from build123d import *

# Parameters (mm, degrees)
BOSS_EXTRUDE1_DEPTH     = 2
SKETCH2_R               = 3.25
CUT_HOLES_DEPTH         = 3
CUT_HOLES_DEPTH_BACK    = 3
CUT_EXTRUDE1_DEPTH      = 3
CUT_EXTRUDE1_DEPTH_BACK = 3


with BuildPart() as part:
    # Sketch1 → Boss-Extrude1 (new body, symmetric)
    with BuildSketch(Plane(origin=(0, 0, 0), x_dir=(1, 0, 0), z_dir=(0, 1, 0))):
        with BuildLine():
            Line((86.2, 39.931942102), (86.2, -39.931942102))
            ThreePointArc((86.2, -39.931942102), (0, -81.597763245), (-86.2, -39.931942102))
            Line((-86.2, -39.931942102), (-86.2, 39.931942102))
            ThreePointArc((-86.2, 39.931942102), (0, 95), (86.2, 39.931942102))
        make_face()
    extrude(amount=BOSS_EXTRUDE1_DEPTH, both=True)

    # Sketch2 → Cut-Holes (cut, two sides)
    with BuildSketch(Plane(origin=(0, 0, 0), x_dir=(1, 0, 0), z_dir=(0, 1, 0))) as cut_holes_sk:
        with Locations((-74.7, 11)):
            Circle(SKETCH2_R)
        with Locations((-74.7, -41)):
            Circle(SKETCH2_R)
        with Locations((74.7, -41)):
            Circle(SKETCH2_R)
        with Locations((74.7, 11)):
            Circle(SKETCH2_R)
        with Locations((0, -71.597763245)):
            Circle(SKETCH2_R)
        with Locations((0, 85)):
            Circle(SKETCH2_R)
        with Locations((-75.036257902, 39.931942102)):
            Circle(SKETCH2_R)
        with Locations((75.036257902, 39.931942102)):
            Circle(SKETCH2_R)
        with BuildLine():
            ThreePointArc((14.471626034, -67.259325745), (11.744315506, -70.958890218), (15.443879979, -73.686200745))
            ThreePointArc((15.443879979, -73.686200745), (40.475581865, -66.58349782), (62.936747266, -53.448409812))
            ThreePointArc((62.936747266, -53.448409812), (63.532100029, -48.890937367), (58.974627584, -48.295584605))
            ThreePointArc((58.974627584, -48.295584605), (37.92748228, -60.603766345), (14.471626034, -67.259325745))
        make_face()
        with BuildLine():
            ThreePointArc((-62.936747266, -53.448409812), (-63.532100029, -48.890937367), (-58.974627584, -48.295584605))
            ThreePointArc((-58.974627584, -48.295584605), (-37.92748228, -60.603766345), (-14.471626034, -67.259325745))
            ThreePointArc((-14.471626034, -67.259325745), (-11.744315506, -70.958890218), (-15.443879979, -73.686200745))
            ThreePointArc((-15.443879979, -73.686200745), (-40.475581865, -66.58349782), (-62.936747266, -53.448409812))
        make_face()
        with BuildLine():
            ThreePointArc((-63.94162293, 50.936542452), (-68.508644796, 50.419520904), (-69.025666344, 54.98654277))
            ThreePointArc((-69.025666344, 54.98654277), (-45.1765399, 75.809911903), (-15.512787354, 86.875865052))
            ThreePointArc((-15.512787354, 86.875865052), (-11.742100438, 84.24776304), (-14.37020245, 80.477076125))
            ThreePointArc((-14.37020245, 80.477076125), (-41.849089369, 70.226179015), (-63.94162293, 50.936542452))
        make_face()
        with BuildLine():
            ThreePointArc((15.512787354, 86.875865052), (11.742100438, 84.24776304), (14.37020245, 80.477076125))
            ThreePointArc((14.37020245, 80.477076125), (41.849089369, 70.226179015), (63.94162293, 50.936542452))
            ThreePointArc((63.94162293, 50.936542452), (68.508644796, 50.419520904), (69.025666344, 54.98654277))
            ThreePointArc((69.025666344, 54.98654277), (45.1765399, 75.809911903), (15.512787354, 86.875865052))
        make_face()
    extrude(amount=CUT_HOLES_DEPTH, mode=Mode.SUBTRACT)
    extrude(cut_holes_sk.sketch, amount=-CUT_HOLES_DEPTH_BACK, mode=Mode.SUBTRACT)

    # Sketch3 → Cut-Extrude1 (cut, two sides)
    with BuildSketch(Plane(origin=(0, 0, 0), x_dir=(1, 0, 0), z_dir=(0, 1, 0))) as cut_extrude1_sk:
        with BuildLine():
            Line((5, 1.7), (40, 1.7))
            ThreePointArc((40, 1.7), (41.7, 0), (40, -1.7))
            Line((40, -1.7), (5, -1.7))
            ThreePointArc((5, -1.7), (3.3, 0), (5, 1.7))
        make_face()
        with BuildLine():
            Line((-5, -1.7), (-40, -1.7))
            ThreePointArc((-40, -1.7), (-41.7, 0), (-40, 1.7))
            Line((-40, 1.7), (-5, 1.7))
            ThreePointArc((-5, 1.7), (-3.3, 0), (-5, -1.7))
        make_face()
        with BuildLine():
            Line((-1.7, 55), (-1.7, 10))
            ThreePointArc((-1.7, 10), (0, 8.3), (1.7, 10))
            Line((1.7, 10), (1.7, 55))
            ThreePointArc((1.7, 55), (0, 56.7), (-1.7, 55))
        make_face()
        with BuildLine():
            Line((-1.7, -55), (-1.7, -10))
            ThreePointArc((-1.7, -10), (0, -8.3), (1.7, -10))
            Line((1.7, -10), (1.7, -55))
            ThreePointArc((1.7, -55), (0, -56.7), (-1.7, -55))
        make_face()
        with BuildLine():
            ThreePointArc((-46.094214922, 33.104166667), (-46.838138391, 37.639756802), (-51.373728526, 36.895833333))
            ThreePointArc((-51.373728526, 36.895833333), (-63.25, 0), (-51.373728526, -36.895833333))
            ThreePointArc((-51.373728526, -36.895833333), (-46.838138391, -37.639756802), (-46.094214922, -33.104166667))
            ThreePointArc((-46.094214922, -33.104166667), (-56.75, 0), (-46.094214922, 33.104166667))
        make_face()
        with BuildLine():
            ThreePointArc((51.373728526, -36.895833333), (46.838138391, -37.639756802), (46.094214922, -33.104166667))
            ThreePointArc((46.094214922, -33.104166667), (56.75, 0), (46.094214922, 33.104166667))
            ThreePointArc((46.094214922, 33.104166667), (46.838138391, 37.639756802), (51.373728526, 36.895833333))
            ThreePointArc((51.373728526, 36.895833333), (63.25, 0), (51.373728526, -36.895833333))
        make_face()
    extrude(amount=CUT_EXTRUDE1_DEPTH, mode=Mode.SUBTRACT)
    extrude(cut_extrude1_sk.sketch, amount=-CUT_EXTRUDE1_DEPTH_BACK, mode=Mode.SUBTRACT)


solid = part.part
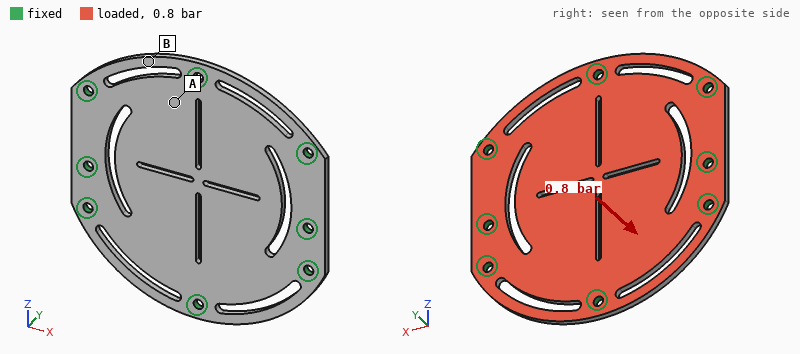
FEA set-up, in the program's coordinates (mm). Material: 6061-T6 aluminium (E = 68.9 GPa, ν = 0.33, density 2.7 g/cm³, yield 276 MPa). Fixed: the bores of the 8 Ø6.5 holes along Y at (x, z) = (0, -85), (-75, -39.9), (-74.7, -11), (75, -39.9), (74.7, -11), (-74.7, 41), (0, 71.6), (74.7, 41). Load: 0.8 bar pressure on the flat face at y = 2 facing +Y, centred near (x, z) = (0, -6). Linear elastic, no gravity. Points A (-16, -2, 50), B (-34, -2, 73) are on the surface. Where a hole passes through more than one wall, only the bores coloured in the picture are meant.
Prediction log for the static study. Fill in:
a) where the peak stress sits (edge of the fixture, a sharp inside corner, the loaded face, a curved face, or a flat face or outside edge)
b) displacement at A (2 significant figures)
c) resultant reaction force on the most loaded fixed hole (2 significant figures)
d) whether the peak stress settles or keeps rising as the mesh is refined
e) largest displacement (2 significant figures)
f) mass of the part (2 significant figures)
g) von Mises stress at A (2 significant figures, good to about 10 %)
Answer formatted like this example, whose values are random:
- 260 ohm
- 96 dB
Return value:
- edge of the fixture
- 0.080 mm
- 350 N
- keeps rising
- 0.35 mm
- 240 g
- 15 MPa
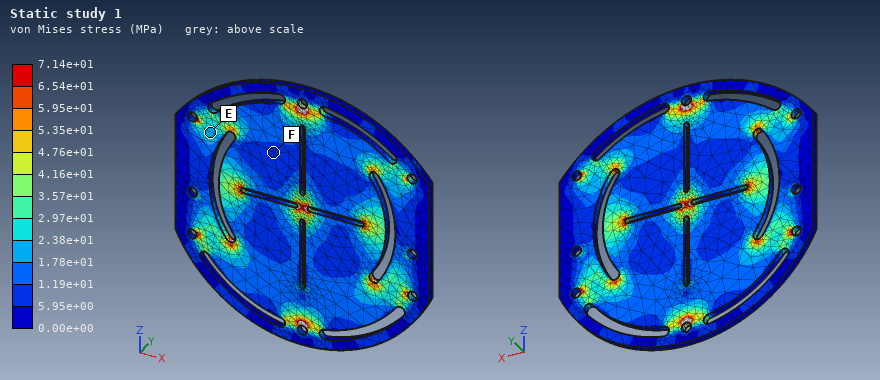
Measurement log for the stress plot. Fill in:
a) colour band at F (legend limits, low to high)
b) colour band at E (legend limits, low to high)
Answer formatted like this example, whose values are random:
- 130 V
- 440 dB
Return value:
- 5.95e+00 to 1.19e+01 MPa
- 1.78e+01 to 2.38e+01 MPa
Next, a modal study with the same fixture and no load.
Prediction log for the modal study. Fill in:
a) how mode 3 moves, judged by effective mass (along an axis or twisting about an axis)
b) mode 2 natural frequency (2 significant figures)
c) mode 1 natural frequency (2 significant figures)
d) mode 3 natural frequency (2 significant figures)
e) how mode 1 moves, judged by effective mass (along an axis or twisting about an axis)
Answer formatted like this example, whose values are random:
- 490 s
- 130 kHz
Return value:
- twisting about X
- 1600 Hz
- 920 Hz
- 2200 Hz
- along Y
